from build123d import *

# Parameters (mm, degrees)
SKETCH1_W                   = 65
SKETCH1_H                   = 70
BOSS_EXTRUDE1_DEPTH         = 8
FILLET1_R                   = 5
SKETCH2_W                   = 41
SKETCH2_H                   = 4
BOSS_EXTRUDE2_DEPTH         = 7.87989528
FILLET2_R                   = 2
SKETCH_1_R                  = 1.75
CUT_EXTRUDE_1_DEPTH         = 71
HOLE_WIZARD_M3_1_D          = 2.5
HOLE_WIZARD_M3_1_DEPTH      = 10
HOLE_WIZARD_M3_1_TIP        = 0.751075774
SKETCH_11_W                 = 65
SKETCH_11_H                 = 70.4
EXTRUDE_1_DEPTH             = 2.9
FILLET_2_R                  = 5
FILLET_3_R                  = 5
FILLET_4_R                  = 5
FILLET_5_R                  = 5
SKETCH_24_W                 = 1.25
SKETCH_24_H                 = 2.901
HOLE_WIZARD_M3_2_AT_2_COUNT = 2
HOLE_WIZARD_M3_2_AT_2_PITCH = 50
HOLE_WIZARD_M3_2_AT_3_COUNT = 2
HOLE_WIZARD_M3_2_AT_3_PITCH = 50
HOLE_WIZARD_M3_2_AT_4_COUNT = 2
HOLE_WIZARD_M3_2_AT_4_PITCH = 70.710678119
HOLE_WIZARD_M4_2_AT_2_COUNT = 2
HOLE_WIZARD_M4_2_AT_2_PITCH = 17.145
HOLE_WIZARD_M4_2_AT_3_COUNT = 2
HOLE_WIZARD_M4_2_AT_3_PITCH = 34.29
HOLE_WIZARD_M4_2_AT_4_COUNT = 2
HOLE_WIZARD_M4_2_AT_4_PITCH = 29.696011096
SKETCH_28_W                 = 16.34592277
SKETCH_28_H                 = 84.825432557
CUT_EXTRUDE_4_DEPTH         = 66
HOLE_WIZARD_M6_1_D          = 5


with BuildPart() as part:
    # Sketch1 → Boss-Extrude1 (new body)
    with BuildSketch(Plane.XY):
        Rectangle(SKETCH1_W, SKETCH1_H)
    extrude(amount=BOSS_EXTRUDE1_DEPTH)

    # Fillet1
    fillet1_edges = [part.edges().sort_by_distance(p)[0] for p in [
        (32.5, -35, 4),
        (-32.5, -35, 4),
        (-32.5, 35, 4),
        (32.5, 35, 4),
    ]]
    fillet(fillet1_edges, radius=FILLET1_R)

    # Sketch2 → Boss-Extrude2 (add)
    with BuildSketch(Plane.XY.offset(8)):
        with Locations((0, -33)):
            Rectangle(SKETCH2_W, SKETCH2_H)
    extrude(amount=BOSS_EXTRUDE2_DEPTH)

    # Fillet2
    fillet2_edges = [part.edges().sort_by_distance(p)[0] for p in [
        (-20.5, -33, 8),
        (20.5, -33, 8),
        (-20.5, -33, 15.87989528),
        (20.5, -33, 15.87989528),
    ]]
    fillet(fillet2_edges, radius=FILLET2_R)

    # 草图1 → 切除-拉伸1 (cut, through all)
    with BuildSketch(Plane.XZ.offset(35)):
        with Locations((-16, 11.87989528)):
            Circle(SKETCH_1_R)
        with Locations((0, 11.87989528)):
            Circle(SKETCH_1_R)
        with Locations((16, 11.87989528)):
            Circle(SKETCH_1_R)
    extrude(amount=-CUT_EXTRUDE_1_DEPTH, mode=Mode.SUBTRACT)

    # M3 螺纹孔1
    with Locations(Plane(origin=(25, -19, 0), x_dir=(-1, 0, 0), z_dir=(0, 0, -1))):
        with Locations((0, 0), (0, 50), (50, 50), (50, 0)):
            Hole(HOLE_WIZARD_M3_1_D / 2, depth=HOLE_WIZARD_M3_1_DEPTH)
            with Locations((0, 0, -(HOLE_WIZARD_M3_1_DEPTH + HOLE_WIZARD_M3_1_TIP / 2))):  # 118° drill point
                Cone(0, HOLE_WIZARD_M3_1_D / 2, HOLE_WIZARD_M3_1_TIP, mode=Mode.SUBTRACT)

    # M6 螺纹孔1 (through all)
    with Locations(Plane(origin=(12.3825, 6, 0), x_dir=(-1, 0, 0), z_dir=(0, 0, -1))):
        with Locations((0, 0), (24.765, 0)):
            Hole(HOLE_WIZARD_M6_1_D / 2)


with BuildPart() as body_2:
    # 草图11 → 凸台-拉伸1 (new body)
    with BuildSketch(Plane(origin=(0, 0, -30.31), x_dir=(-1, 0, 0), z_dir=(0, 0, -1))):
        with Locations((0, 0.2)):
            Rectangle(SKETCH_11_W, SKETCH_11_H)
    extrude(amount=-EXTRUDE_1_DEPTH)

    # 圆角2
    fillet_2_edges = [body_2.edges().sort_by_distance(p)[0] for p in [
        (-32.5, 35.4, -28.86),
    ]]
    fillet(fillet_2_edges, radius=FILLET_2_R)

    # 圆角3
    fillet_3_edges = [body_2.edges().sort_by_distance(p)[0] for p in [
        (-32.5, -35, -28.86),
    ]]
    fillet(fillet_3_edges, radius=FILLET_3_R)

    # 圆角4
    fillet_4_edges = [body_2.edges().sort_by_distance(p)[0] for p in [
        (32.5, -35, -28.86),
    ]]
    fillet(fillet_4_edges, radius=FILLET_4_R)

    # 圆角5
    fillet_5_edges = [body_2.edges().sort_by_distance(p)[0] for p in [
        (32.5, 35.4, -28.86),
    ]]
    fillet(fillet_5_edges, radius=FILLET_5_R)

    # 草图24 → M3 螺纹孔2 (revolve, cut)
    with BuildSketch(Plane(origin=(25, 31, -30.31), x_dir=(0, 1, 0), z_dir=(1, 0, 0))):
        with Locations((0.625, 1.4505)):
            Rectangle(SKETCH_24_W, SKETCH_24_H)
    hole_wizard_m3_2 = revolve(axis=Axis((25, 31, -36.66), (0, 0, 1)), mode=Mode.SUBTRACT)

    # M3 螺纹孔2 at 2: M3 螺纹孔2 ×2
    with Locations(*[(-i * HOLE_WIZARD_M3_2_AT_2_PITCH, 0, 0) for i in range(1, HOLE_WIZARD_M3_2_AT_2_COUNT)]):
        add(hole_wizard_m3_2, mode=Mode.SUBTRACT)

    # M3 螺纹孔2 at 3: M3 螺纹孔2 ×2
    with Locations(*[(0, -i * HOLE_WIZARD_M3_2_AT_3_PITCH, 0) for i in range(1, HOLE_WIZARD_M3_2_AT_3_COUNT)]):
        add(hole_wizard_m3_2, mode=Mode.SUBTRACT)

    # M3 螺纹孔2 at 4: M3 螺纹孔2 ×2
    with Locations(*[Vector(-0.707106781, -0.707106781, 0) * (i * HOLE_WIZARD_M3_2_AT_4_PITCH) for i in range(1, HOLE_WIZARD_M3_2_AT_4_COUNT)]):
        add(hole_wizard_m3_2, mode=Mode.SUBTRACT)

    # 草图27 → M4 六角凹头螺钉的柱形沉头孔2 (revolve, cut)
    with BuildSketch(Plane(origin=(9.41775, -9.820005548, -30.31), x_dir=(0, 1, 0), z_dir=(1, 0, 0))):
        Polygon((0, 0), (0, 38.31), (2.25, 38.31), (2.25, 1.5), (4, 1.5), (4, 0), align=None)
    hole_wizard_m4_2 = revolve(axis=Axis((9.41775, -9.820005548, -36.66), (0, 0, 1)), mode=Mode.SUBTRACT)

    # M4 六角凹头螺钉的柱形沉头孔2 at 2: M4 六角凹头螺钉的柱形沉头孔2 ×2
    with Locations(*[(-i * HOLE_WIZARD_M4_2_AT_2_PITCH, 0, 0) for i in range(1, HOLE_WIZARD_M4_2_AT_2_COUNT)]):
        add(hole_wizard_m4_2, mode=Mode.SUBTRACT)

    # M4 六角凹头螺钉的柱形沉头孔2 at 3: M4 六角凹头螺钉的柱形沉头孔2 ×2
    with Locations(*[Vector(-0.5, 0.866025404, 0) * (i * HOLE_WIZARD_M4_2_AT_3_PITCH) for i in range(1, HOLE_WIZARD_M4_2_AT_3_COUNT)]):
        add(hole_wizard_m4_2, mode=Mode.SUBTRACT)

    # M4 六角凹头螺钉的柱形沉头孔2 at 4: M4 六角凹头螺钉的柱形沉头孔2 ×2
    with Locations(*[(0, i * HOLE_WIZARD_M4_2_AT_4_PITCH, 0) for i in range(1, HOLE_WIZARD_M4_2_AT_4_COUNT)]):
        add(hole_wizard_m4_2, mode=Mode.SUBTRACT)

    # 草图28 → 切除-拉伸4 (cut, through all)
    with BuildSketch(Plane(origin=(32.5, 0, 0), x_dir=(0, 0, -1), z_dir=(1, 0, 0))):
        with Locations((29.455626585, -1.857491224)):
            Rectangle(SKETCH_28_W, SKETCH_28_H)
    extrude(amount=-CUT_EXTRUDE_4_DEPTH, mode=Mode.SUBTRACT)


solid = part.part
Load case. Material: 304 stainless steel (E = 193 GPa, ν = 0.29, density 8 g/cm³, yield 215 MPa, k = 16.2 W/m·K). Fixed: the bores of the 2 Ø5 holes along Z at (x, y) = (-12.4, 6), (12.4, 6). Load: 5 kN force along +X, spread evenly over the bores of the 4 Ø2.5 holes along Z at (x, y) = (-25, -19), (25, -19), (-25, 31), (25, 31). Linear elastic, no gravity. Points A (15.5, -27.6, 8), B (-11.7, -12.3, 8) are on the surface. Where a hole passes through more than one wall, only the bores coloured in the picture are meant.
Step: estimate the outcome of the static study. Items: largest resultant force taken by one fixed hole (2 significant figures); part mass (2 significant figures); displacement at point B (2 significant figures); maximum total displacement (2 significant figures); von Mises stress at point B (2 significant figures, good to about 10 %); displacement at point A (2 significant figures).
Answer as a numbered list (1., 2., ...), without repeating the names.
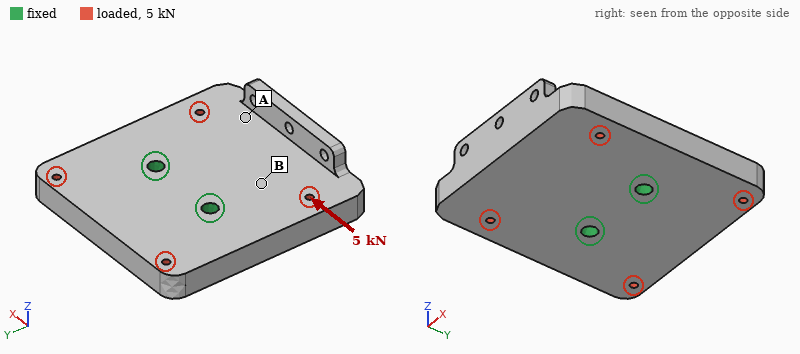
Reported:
1. 2.5 kN
2. 300 g
3. 1.7 µm
4. 3.5 µm
5. 9.3 MPa
6. 2.6 µm
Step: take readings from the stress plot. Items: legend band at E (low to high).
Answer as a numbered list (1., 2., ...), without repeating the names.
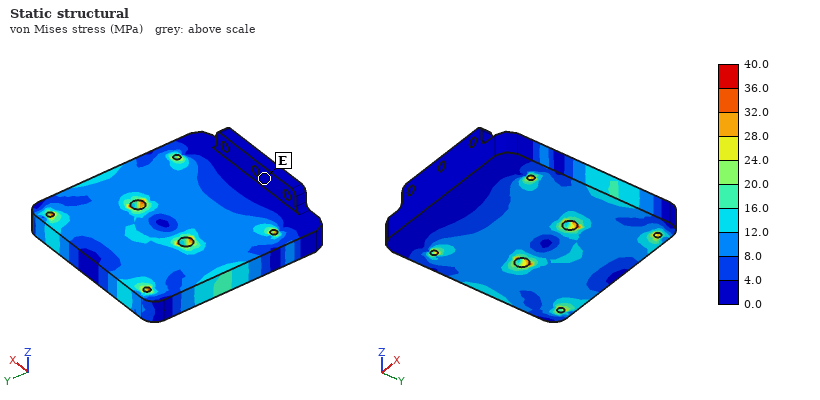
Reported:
1. 0.0 to 4.0 MPa
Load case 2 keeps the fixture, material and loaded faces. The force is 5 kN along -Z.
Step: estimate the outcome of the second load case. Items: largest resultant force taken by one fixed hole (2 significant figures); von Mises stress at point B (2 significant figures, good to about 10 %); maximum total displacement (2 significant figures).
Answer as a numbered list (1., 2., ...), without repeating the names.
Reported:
1. 2.5 kN
2. 24 MPa
3. 45 µm
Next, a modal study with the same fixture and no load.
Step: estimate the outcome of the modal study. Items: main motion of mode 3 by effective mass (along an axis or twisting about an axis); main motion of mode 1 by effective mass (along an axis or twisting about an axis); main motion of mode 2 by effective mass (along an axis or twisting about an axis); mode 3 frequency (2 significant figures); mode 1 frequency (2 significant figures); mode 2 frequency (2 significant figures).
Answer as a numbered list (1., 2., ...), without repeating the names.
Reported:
1. along Z
2. along Z
3. twisting about Y
4. 6700 Hz
5. 3100 Hz
6. 5200 Hz
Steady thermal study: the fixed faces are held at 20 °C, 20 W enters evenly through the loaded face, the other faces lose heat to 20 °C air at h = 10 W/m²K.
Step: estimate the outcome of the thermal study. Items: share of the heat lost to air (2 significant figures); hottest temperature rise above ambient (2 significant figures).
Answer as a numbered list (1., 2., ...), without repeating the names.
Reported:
1. 16 %
2. 55 K
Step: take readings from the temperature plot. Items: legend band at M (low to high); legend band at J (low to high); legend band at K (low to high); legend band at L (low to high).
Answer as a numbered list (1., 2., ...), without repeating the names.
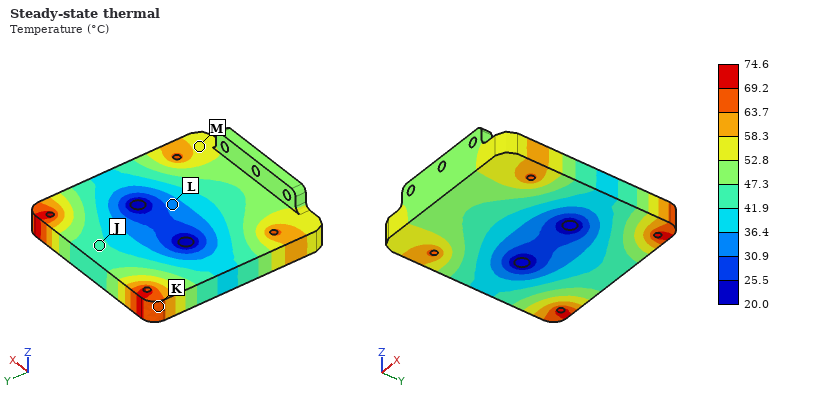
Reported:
1. 52.8 to 58.3 °C
2. 41.9 to 47.3 °C
3. 63.7 to 69.2 °C
4. 30.9 to 36.4 °C
